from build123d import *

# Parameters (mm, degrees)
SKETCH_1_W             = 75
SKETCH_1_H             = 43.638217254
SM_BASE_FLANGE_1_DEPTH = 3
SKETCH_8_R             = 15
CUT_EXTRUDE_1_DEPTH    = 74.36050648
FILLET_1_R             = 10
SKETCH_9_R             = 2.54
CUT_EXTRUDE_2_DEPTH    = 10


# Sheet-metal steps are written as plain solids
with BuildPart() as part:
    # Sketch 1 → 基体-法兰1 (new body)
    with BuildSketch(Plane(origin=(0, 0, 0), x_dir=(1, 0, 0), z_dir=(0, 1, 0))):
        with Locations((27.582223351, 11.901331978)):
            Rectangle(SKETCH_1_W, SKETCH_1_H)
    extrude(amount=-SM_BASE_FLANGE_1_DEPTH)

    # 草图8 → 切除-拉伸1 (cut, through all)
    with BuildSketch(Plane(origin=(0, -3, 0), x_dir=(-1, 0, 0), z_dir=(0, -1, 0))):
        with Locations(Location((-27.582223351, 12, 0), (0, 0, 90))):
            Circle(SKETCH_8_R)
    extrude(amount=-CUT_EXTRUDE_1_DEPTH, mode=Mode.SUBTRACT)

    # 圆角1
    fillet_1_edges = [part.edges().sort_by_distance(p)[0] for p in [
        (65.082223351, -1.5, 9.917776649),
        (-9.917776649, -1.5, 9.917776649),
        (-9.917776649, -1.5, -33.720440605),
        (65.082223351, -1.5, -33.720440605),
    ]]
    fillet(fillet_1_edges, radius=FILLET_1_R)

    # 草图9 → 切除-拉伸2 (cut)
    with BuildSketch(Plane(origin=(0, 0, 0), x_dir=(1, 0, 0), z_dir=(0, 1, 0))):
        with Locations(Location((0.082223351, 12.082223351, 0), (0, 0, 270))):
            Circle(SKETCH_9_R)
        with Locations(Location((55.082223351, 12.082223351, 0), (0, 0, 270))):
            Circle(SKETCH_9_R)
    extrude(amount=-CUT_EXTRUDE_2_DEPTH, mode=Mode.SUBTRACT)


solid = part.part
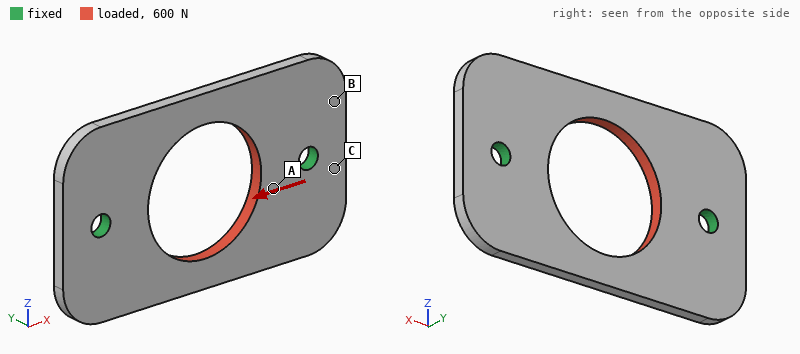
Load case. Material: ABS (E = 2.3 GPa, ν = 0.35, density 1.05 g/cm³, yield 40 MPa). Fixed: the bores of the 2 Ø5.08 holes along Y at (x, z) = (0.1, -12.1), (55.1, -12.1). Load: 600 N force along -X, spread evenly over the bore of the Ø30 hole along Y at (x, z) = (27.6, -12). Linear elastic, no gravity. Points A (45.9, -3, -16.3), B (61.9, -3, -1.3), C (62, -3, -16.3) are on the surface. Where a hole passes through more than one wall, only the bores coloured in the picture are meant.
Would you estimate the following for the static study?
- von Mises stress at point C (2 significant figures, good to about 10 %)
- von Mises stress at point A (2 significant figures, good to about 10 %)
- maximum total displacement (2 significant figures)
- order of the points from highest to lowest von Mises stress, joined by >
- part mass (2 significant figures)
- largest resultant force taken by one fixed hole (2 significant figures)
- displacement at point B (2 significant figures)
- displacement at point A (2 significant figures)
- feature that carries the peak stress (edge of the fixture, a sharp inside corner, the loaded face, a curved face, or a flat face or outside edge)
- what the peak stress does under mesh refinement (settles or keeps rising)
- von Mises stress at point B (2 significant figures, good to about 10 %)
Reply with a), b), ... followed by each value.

a) 3.3 MPa
b) 5.1 MPa
c) 74 µm
d) A > C > B
e) 7.7 g
f) 300 N
g) 31 µm
h) 23 µm
i) edge of the fixture
j) keeps rising
k) 1.5 MPa
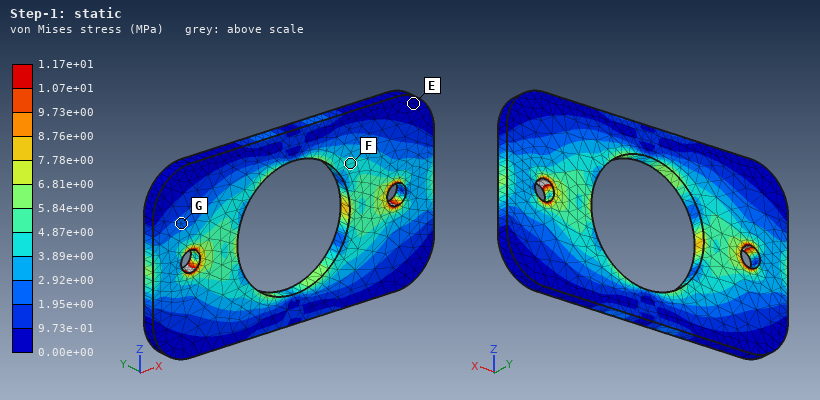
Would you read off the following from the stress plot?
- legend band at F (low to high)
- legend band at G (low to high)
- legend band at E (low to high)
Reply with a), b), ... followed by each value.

a) 3.89e+00 to 4.87e+00 MPa
b) 1.95e+00 to 2.92e+00 MPa
c) 0.00e+00 to 9.73e-01 MPa
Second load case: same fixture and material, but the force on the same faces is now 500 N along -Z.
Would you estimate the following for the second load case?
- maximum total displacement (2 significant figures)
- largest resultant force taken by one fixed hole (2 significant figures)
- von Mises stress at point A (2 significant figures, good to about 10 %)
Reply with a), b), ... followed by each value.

a) 0.11 mm
b) 250 N
c) 5.1 MPa
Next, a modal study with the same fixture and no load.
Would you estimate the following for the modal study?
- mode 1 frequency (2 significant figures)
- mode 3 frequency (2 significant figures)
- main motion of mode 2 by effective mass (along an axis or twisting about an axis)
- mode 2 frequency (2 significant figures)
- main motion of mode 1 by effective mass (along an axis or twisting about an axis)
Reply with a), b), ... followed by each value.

a) 1000 Hz
b) 1800 Hz
c) along Y
d) 1200 Hz
e) twisting about X
